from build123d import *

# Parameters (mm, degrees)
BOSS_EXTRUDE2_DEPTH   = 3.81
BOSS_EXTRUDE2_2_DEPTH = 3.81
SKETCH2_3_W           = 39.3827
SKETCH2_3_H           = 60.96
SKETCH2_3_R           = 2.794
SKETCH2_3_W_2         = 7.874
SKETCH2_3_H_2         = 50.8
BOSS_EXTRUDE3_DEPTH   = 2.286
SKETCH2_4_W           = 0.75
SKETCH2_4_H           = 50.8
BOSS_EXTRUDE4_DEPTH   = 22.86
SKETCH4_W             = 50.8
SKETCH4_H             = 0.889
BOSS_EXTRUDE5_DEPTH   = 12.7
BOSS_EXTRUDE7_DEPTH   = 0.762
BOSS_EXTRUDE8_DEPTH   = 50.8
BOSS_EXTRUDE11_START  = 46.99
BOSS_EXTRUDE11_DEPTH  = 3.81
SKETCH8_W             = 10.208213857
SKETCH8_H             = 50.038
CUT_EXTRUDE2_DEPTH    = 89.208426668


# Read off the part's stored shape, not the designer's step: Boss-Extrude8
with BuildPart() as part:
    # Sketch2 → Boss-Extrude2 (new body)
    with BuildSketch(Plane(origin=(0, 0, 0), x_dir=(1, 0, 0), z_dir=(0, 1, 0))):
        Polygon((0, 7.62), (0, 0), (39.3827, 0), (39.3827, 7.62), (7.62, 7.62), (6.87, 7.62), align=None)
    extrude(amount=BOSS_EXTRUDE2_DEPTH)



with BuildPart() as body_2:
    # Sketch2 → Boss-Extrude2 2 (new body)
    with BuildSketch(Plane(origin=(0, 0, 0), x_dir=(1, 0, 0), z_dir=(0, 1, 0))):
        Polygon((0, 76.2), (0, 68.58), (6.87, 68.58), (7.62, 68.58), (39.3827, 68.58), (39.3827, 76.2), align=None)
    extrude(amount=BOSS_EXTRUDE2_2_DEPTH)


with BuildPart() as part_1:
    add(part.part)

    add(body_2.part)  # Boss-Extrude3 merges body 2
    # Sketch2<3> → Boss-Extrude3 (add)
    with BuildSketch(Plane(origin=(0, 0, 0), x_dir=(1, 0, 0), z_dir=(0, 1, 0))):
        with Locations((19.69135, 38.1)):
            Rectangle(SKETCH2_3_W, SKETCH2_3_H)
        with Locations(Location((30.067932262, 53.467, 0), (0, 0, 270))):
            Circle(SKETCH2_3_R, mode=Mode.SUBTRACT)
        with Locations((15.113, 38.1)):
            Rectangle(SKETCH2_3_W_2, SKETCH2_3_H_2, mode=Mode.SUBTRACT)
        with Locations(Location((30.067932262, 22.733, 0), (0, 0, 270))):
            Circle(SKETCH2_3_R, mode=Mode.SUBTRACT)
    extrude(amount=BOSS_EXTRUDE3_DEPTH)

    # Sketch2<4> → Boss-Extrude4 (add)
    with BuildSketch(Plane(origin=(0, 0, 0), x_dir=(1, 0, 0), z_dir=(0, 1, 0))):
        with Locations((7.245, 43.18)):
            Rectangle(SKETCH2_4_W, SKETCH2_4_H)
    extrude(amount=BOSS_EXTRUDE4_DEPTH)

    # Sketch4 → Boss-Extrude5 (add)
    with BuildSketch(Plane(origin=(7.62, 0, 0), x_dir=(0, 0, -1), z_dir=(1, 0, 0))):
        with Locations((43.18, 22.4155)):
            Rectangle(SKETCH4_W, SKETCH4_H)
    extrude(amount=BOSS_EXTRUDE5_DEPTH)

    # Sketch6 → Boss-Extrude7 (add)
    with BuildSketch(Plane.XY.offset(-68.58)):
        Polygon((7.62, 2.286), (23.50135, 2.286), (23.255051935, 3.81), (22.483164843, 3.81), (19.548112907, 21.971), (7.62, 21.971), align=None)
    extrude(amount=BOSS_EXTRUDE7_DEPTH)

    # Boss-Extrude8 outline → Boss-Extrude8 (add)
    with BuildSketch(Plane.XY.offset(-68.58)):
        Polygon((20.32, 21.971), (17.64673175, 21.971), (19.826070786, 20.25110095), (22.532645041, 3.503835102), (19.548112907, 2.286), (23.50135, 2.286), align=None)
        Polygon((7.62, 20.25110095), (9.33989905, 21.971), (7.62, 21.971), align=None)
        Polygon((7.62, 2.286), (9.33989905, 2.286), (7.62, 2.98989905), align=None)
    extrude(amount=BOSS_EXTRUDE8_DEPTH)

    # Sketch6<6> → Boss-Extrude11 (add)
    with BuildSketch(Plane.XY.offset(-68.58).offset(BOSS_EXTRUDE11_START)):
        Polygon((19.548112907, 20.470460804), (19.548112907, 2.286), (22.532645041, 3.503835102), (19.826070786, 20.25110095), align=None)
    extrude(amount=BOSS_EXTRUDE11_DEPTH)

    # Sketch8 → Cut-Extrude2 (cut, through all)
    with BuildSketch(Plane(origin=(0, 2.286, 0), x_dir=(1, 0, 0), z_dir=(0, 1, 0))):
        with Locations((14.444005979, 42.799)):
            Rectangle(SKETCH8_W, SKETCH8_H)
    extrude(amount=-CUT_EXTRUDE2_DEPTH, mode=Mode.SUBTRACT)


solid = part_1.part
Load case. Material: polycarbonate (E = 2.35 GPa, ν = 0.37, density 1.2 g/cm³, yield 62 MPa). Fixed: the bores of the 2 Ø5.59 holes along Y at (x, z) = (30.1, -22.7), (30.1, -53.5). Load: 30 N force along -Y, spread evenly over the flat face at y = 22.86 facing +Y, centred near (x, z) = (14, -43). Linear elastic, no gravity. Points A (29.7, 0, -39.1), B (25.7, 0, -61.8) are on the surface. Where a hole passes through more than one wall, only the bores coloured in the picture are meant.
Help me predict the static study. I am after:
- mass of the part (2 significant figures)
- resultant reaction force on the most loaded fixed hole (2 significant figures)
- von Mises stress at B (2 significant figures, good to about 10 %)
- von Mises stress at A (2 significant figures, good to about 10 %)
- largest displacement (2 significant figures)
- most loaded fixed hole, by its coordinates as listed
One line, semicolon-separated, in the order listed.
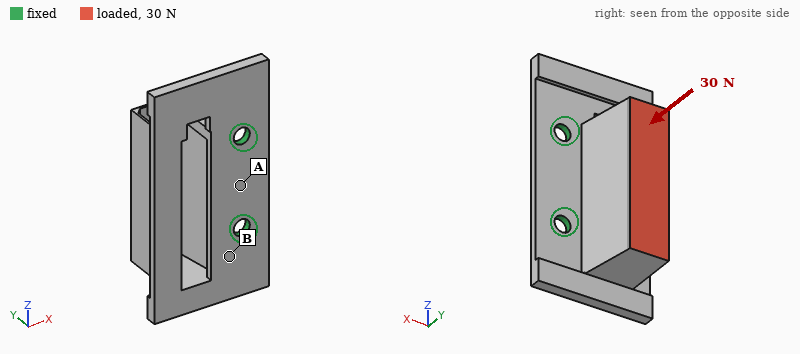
11 g; 22 N; 4.5 MPa; 1.3 MPa; 0.93 mm; (30.1, -53.5)
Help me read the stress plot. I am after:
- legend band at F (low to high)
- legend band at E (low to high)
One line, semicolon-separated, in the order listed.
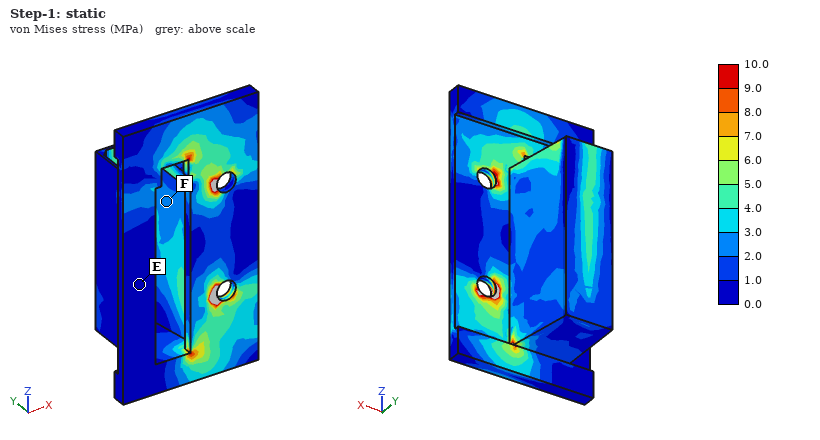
2.0 to 3.0 MPa; 0.0 to 1.0 MPa
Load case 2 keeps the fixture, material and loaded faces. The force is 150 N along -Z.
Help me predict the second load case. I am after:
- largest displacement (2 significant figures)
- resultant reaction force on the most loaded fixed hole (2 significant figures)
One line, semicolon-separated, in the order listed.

0.82 mm; 140 N
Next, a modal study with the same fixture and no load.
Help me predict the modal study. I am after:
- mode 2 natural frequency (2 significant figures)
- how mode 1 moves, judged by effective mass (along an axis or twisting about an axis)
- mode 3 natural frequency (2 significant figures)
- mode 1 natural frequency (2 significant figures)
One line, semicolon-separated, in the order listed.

740 Hz; along Y; 1000 Hz; 350 Hz
